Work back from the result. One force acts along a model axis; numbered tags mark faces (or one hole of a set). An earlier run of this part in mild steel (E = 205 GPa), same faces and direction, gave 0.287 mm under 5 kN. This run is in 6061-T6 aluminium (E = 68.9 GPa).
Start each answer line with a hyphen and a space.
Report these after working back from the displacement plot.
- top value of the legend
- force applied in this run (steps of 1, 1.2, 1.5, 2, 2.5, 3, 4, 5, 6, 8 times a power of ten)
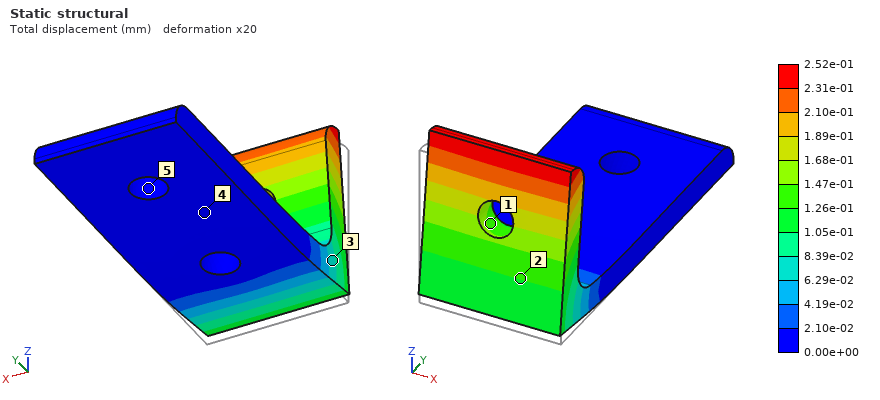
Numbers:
- 2.52e-01 mm
- 1.5 kN
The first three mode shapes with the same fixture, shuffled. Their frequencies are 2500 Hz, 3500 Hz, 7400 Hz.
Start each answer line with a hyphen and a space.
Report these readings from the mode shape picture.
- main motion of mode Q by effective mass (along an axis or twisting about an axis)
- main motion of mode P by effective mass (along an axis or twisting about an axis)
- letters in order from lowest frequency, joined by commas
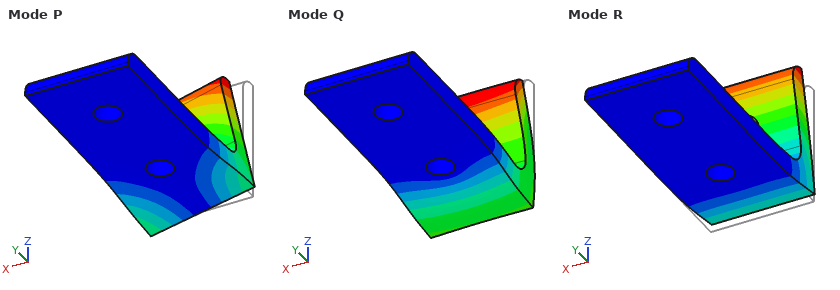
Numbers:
- along Z
- along X
- R, P, Q
